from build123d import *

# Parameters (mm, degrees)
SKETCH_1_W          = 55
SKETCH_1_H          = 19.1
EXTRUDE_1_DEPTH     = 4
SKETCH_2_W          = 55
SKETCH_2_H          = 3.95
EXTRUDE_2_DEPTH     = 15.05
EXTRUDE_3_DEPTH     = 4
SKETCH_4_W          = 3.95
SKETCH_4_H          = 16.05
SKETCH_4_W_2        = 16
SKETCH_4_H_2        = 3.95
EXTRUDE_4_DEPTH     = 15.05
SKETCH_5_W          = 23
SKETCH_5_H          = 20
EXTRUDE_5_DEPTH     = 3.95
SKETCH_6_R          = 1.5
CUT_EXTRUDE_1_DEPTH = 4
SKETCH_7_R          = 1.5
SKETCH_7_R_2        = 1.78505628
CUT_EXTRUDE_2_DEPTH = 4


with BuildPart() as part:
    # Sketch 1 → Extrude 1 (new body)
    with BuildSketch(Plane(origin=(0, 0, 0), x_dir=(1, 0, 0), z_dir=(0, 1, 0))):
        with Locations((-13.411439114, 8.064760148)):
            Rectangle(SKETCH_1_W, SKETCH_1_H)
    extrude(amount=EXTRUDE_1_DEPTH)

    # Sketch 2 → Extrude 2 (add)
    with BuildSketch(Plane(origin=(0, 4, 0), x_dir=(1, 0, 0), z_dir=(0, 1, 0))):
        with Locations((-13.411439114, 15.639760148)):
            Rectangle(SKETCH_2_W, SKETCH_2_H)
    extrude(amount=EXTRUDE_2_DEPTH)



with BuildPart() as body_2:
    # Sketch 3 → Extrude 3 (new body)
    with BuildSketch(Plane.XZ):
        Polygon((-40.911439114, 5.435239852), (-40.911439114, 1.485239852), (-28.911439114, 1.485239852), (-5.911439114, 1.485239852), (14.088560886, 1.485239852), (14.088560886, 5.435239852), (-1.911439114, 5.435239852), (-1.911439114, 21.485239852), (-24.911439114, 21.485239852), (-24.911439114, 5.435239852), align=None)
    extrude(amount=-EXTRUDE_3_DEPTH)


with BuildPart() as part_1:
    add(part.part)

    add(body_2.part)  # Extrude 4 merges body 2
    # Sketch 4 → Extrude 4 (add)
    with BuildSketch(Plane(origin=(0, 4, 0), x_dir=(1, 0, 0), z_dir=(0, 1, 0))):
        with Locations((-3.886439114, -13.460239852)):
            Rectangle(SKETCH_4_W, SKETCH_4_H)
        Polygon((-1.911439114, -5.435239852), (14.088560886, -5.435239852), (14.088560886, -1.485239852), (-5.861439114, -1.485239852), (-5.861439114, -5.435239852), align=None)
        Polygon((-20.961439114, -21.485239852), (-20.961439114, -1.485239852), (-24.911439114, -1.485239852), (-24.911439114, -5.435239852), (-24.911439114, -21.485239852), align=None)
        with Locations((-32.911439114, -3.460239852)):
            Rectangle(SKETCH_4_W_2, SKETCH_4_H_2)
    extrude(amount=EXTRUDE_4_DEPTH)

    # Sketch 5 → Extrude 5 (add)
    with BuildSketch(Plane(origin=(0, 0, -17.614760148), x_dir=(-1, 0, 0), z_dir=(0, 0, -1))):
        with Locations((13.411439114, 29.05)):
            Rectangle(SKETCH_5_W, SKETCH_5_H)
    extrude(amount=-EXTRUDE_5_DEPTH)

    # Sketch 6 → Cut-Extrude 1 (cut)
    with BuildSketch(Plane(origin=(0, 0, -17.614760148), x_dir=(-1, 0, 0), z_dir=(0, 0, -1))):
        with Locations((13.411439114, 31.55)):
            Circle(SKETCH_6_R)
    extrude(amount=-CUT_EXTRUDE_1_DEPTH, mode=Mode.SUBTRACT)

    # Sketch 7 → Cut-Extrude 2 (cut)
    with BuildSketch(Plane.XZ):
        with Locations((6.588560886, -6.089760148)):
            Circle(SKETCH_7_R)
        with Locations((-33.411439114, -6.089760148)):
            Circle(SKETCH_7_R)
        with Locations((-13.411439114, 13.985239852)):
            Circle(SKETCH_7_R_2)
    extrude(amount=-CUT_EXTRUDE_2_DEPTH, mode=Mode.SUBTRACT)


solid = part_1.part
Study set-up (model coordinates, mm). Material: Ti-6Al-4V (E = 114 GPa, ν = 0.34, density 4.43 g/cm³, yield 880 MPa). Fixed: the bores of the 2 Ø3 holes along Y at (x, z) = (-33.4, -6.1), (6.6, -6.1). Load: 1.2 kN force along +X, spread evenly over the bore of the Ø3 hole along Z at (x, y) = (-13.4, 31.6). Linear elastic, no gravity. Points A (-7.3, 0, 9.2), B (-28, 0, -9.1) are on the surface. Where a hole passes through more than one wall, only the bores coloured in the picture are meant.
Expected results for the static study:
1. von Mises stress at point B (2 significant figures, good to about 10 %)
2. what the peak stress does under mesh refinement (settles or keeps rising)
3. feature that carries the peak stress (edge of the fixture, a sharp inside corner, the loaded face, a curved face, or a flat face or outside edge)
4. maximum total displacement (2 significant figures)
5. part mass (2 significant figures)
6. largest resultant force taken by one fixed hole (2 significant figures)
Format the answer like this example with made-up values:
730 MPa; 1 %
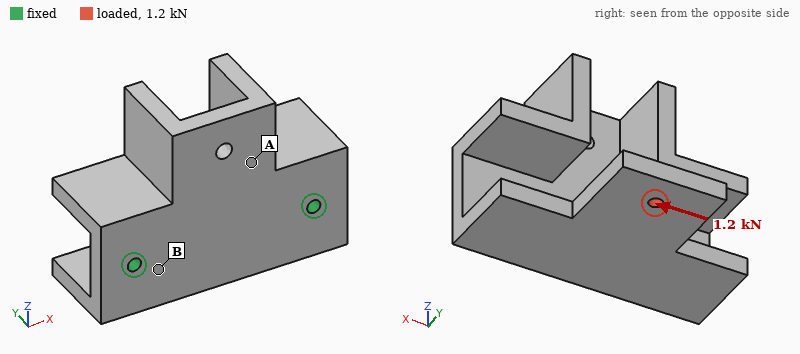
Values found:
36 MPa; keeps rising; edge of the fixture; 62 µm; 70 g; 1.1 kN
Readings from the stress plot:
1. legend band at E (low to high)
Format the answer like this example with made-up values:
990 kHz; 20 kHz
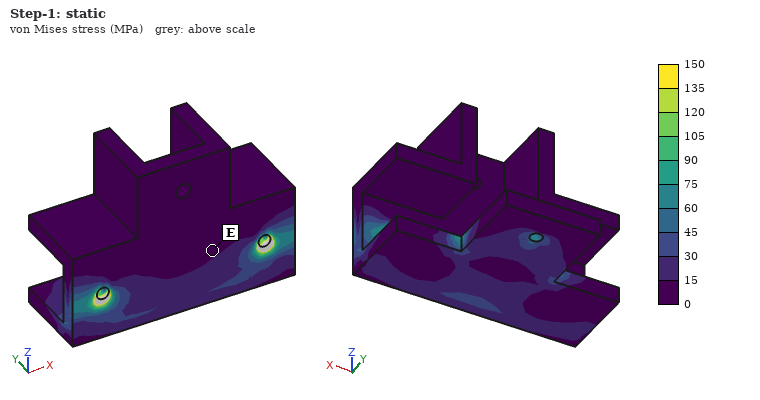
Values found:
0 to 15 MPa
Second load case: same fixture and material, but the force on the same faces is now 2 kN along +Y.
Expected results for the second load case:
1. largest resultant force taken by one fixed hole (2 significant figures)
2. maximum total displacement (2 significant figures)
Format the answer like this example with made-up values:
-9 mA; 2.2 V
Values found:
1.0 kN; 0.16 mm
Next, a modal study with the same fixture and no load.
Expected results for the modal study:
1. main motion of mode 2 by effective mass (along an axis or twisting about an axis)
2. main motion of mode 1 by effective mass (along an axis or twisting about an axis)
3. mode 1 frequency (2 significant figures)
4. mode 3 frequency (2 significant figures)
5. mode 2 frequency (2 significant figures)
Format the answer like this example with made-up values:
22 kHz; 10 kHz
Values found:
along Y; along Z; 2100 Hz; 6300 Hz; 3000 Hz
